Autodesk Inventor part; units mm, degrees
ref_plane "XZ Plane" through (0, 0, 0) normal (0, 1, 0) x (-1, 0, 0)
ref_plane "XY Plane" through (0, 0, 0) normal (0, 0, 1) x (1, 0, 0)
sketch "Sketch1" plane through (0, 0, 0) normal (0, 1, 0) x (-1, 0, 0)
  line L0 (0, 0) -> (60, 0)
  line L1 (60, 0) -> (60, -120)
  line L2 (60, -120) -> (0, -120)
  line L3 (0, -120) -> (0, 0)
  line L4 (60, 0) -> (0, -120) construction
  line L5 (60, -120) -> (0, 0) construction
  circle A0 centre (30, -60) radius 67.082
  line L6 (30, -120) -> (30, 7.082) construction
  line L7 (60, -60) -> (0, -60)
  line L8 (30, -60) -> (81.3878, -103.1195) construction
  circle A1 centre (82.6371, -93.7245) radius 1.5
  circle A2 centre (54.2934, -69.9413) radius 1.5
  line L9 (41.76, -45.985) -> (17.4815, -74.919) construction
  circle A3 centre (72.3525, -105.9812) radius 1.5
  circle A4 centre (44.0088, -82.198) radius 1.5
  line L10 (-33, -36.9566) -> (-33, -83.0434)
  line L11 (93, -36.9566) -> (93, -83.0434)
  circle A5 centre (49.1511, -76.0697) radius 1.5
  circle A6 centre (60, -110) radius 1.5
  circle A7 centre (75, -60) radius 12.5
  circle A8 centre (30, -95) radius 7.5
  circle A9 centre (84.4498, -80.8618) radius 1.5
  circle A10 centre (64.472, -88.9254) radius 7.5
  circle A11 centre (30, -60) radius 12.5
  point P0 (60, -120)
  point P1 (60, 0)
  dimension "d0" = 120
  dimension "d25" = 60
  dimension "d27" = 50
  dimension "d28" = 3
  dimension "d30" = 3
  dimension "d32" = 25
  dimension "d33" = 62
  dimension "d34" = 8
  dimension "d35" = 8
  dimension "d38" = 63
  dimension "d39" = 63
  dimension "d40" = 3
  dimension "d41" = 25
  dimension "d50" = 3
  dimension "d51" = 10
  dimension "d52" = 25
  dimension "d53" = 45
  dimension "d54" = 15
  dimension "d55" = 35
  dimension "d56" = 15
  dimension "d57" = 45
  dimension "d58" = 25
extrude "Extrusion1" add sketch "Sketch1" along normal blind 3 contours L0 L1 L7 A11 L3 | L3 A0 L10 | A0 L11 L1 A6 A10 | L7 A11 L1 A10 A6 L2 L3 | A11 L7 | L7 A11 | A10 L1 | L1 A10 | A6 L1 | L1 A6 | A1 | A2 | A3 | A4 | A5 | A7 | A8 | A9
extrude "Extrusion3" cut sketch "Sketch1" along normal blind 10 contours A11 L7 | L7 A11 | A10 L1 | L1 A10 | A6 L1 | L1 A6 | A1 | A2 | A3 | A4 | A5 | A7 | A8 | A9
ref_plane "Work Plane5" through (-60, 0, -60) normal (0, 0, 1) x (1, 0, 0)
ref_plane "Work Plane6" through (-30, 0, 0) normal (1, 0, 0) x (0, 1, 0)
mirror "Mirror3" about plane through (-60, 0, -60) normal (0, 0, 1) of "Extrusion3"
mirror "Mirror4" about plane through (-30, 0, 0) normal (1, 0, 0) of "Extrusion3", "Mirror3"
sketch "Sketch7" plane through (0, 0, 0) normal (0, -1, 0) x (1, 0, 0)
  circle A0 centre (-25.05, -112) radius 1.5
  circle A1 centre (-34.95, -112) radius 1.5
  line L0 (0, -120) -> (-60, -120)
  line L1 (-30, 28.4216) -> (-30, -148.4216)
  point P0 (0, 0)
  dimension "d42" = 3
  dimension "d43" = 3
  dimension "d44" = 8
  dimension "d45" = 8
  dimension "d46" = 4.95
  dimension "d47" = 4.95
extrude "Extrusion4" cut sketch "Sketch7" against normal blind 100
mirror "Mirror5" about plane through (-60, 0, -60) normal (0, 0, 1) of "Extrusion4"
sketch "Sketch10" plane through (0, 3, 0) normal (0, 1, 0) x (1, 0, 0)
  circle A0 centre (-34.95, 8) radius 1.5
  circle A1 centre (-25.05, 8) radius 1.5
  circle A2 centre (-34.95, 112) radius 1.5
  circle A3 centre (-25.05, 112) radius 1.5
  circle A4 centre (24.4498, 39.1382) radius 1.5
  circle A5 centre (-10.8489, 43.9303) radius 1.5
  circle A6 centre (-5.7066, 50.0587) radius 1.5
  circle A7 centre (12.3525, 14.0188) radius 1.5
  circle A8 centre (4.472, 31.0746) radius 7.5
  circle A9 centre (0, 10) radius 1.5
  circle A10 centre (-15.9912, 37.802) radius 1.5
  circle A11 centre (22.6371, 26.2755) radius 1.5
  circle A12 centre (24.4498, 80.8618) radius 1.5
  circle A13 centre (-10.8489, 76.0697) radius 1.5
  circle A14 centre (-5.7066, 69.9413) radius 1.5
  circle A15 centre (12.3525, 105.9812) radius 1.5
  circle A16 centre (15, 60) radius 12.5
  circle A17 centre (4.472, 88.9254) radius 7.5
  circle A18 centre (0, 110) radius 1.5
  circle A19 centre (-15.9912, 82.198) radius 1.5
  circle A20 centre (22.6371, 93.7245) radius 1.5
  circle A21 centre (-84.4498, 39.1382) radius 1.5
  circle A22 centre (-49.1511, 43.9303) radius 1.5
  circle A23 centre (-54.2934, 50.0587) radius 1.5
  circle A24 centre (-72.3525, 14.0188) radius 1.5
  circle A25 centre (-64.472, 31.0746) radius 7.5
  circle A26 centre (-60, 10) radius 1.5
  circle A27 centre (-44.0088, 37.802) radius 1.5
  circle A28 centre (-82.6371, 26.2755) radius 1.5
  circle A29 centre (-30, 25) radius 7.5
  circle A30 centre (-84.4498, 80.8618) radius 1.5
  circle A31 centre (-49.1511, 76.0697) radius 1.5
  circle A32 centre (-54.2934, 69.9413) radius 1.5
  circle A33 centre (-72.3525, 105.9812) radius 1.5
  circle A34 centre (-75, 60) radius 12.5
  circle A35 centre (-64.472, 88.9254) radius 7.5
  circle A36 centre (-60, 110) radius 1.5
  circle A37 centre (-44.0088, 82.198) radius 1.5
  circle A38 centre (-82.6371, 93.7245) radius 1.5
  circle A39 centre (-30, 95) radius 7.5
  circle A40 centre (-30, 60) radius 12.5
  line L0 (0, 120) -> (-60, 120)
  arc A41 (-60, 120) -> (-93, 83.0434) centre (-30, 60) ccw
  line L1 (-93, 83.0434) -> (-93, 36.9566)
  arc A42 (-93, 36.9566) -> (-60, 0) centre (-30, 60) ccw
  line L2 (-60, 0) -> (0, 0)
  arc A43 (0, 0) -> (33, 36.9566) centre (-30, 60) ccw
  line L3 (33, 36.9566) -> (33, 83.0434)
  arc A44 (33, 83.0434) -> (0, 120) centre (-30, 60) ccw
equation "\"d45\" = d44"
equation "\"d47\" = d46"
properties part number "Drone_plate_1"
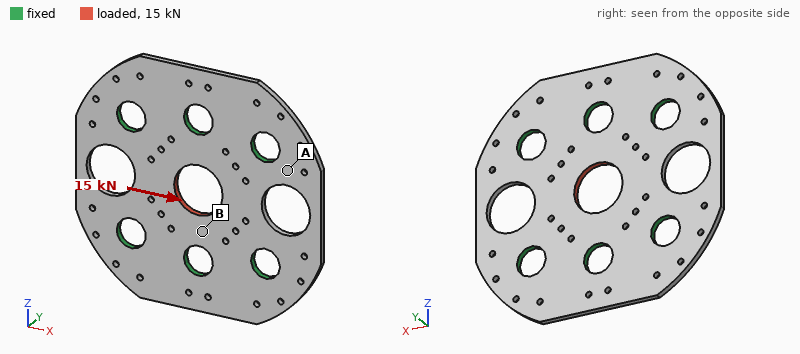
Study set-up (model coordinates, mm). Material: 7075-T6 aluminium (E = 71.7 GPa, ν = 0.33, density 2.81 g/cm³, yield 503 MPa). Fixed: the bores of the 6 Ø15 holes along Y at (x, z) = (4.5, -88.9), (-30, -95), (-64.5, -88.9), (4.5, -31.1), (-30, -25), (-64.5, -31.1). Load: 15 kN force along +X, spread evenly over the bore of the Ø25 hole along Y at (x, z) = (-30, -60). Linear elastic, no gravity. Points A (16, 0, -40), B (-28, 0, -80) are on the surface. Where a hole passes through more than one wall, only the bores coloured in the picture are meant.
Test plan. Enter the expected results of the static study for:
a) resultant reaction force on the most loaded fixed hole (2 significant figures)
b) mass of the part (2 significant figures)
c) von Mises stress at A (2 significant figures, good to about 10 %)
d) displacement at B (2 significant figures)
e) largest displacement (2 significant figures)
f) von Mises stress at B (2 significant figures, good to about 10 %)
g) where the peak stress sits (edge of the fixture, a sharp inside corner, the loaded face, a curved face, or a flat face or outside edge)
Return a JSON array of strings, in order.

["3.2 kN", "89 g", "19 MPa", "11 µm", "29 µm", "59 MPa", "a curved face"]
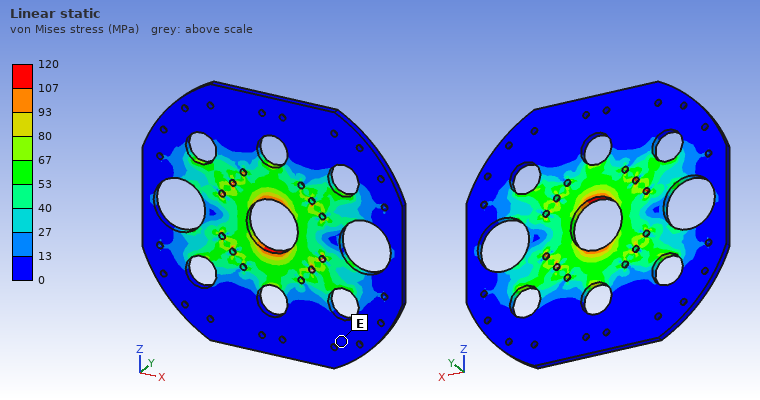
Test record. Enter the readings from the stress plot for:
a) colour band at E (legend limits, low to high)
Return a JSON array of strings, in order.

["0 to 13 MPa"]
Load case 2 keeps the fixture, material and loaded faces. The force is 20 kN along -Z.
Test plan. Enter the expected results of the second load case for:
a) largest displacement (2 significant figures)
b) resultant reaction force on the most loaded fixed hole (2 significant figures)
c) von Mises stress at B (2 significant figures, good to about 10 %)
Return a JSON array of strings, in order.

["27 µm", "6.0 kN", "93 MPa"]
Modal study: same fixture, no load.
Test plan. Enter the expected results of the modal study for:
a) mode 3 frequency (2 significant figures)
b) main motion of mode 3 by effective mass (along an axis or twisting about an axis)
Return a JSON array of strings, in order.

["5400 Hz", "twisting about X"]
